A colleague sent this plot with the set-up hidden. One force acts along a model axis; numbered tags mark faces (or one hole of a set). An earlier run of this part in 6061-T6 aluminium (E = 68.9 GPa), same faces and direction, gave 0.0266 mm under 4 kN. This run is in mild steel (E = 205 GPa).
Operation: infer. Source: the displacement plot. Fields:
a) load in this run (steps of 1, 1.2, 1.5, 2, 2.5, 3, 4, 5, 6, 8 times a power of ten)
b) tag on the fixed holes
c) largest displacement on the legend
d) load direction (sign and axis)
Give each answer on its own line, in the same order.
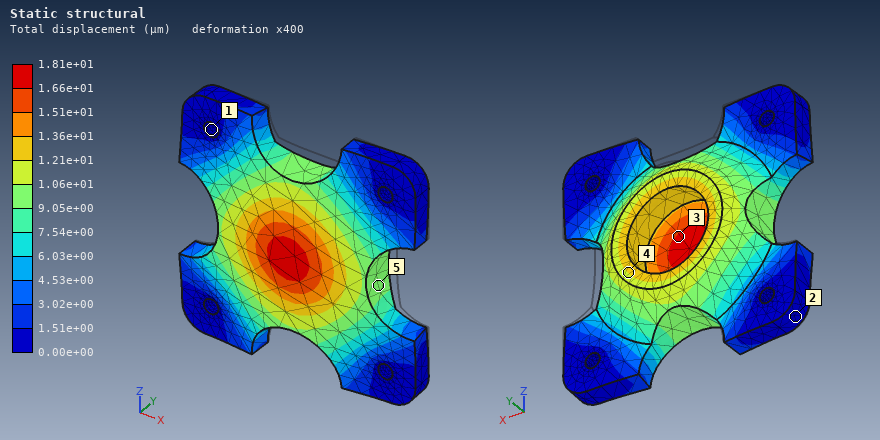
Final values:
8 kN
1
1.81e+01 µm
-Y
